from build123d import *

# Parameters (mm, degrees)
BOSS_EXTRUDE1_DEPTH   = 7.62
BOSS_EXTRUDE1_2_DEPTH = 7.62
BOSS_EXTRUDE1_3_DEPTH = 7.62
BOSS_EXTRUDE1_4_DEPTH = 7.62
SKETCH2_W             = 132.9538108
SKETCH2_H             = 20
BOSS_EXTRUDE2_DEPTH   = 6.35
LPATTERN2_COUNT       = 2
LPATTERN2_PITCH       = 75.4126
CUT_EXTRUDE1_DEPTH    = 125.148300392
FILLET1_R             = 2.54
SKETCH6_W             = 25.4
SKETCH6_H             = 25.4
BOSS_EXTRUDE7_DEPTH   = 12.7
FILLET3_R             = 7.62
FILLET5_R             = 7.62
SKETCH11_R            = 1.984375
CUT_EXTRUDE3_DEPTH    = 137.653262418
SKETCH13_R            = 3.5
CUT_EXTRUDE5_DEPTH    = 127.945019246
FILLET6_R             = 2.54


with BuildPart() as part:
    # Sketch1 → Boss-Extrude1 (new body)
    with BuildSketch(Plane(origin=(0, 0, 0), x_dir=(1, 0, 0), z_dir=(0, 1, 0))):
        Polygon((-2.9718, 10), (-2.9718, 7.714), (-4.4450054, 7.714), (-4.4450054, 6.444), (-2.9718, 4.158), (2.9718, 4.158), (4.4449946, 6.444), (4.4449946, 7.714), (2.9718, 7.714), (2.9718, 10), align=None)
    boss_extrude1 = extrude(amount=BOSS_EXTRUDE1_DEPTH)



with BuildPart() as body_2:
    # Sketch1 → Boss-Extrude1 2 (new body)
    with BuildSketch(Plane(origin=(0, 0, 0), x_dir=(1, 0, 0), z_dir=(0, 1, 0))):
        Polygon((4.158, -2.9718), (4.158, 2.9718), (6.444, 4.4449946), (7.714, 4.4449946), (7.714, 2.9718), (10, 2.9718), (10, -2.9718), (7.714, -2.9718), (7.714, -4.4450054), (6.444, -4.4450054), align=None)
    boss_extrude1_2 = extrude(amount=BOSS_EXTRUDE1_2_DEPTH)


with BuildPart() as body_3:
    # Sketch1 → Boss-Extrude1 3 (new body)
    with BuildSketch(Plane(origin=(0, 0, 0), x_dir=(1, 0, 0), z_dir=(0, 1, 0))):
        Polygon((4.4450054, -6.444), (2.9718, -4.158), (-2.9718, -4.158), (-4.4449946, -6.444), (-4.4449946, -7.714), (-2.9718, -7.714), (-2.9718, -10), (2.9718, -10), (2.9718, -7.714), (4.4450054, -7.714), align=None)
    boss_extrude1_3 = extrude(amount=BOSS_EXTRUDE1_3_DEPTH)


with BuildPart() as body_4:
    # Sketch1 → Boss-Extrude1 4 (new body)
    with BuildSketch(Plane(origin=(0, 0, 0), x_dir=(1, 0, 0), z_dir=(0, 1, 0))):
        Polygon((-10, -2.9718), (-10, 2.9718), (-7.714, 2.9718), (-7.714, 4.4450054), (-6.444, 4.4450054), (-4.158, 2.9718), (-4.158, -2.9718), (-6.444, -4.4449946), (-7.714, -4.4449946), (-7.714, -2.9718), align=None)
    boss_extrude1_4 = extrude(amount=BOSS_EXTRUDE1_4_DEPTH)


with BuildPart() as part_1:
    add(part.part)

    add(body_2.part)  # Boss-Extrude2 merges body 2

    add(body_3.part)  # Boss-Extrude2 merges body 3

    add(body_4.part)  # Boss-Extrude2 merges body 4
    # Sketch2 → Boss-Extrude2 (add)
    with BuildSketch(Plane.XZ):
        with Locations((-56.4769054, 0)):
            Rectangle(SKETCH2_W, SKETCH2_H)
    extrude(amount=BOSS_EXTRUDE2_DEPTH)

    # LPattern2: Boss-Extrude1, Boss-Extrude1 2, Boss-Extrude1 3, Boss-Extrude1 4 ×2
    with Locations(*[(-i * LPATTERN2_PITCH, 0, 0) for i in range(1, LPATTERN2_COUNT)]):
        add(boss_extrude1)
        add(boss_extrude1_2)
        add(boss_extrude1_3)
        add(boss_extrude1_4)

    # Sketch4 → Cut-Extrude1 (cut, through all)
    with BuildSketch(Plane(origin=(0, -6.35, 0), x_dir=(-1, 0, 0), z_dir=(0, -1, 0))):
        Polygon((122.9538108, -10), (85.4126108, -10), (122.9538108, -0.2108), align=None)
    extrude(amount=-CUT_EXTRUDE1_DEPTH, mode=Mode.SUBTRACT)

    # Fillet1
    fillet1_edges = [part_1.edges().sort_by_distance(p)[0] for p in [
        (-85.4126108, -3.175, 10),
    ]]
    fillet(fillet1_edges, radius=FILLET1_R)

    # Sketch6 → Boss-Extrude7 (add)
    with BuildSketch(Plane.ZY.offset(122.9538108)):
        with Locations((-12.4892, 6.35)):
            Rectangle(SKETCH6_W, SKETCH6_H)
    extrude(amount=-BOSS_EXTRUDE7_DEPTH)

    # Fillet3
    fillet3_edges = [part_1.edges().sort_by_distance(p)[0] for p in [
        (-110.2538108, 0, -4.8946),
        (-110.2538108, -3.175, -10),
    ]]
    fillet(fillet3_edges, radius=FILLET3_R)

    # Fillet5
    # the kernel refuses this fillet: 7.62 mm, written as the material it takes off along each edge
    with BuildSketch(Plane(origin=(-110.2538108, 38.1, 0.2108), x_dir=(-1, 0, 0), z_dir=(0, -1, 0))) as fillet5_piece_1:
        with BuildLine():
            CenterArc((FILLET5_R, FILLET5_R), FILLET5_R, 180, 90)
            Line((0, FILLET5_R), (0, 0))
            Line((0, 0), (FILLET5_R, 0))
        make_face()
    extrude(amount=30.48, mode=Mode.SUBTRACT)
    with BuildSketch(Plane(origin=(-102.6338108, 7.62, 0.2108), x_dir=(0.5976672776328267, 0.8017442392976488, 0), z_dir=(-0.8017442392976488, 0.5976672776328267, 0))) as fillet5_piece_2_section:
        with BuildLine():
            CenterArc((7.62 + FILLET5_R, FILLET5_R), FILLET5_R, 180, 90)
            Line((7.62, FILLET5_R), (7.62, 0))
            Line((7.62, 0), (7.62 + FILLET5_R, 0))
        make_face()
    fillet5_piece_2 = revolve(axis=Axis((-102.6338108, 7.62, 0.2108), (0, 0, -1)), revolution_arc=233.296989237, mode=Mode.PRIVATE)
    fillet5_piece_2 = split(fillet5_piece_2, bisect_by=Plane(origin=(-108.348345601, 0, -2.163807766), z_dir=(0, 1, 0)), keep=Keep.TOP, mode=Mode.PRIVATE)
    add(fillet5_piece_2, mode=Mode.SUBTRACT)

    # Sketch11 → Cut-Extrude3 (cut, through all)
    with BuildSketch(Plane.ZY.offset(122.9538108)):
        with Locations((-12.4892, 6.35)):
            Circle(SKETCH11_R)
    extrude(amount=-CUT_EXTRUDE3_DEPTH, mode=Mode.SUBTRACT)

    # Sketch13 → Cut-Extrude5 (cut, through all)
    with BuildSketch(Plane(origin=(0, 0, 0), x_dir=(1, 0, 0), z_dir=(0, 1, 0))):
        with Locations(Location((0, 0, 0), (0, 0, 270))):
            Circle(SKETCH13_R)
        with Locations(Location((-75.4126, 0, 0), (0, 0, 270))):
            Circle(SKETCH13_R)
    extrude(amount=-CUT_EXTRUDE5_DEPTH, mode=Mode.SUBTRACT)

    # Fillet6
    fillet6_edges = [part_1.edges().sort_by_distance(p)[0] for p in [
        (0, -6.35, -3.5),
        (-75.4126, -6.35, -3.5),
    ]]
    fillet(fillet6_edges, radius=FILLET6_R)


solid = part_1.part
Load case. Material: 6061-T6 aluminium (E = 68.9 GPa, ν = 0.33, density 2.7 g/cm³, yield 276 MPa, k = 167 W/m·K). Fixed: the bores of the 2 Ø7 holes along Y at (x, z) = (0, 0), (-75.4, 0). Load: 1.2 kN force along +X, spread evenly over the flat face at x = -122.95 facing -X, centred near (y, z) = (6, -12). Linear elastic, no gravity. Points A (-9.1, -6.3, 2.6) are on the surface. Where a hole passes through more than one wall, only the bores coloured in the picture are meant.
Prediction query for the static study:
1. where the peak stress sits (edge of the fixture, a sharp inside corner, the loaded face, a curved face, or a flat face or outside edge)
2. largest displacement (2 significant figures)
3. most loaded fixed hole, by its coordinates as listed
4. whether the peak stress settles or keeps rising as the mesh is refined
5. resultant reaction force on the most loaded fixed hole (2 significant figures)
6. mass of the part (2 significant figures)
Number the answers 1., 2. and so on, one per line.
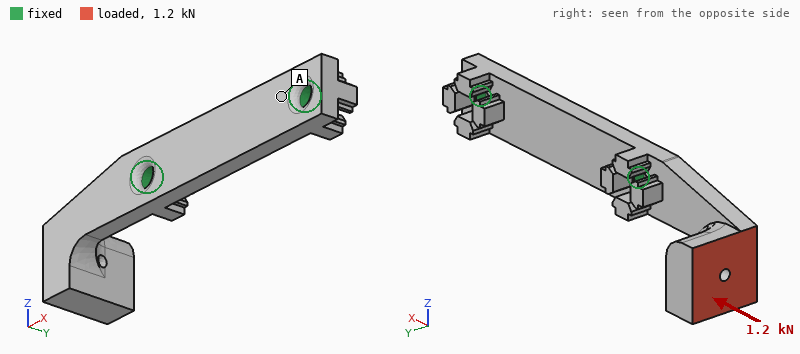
1. edge of the fixture
2. 0.61 mm
3. (-75.4, 0)
4. keeps rising
5. 1.2 kN
6. 67 g
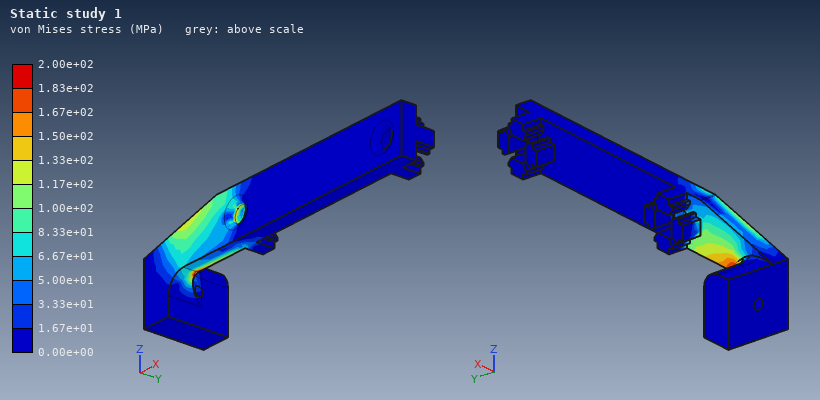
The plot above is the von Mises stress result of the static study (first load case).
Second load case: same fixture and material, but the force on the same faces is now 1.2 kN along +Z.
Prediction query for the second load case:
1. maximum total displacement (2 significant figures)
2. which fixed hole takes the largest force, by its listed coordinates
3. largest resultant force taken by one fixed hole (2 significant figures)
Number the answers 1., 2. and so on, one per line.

1. 0.66 mm
2. (-75.4, 0)
3. 1.5 kN
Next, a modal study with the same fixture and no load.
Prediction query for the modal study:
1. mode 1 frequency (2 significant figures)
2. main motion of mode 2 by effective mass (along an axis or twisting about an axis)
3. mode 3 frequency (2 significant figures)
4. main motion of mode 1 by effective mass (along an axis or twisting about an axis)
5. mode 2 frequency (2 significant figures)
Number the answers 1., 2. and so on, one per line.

1. 980 Hz
2. along Z
3. 3800 Hz
4. along Y
5. 1900 Hz
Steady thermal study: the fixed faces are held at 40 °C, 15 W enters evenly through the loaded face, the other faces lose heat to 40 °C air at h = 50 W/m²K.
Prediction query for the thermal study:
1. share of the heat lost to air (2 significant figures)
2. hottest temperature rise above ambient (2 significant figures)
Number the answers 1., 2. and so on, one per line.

1. 23 %
2. 28 K
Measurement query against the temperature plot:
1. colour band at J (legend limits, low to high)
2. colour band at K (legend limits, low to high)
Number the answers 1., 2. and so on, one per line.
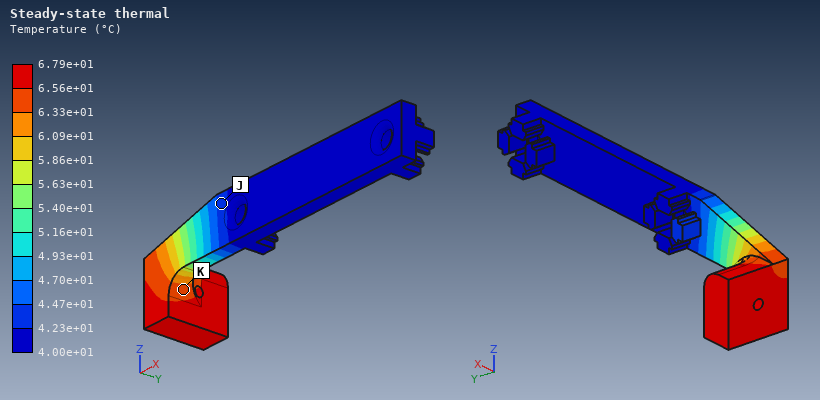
1. 4.23e+01 to 4.47e+01 °C
2. 6.33e+01 to 6.56e+01 °C
